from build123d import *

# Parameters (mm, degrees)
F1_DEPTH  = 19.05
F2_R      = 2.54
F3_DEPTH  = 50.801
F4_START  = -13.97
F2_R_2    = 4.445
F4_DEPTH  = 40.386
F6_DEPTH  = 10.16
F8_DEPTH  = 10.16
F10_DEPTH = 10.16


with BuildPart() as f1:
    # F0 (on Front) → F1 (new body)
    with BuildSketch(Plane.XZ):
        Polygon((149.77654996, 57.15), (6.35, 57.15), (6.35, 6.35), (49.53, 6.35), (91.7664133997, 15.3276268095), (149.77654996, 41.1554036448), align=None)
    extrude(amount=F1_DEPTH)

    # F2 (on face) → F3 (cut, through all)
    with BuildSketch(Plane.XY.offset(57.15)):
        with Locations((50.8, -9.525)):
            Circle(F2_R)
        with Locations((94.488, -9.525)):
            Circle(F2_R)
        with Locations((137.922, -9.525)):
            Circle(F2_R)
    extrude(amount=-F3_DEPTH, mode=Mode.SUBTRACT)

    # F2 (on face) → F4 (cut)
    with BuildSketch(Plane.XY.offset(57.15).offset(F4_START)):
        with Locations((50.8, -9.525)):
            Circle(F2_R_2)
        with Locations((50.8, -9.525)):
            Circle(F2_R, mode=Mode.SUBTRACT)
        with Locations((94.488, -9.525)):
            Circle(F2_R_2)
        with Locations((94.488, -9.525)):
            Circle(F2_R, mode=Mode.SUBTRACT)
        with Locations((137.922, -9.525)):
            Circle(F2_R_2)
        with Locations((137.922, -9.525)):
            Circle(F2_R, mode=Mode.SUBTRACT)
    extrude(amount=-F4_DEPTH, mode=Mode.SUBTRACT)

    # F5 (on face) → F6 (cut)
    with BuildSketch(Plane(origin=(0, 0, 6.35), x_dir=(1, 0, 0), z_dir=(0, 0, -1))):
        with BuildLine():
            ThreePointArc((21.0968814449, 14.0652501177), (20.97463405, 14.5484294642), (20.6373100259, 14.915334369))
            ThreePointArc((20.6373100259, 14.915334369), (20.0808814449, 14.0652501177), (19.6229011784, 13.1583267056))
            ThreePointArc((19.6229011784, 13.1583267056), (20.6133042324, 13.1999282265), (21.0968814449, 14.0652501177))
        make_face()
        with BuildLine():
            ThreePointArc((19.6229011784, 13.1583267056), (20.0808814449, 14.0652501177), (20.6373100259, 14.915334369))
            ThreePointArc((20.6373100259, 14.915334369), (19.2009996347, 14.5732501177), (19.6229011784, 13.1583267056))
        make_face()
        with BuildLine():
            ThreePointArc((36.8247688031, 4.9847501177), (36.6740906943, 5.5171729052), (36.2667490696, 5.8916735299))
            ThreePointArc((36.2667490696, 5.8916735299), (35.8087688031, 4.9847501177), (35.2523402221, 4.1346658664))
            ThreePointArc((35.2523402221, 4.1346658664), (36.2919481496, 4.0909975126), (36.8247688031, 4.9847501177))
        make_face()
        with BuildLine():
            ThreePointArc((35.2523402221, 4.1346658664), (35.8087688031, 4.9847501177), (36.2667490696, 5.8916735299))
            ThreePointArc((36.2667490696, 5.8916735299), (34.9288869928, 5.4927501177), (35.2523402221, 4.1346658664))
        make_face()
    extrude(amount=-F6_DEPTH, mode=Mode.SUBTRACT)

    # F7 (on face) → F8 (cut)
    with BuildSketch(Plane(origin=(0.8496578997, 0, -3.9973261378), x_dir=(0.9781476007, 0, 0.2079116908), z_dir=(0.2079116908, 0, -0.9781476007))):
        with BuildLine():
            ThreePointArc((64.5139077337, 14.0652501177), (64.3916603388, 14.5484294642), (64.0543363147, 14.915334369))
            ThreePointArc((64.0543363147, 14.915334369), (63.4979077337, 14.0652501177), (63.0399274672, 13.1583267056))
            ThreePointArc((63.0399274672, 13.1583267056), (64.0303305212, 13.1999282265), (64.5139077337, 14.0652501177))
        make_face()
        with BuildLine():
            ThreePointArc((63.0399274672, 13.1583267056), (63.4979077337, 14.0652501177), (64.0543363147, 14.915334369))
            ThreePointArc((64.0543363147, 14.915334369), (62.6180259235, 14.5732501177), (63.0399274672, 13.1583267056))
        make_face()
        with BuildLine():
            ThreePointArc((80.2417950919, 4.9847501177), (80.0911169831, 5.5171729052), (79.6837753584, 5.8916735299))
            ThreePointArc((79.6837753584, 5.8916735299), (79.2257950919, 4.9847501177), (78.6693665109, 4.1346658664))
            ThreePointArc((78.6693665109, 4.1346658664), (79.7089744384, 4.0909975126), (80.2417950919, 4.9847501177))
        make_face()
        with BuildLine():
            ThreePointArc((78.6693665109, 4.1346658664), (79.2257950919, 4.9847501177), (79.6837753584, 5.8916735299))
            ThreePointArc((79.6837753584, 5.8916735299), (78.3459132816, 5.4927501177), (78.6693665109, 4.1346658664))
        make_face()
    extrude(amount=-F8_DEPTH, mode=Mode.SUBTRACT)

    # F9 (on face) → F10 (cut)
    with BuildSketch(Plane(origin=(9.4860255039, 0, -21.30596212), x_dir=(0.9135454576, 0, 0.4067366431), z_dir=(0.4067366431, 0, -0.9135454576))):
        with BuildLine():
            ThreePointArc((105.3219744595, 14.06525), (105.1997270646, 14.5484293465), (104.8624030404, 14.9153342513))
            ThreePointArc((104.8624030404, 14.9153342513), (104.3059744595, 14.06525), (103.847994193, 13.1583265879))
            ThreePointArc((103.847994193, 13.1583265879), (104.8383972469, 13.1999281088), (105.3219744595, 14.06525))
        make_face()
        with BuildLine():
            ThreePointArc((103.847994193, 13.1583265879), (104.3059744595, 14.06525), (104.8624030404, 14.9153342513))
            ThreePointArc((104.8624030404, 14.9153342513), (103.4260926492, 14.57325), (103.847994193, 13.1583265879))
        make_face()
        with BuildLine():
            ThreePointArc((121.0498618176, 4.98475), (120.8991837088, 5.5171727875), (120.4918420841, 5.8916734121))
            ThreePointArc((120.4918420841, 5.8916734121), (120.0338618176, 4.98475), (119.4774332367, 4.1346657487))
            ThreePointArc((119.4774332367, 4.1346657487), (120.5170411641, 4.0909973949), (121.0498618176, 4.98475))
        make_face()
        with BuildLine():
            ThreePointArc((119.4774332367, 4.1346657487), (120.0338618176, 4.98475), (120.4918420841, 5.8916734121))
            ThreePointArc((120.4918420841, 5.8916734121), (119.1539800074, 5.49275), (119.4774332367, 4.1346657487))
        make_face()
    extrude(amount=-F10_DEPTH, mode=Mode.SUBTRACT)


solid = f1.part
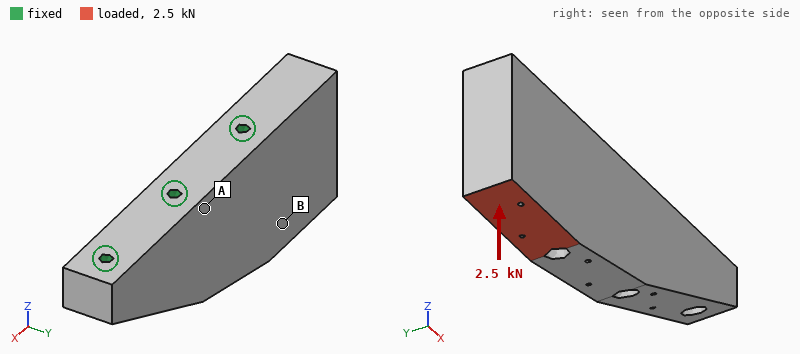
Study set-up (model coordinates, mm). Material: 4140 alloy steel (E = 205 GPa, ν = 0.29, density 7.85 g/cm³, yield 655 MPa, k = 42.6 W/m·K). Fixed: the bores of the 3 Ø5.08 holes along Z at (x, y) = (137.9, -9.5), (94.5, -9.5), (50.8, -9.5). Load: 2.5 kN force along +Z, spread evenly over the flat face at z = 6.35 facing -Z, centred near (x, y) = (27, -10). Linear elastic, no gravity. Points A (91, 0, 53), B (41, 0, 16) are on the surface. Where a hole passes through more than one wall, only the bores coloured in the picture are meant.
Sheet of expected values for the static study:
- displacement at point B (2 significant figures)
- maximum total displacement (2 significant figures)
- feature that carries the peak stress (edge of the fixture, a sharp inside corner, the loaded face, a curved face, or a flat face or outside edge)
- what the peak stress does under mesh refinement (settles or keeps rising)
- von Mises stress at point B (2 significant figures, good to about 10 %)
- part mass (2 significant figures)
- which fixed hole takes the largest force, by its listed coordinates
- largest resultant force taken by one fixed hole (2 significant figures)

2.6 µm
5.6 µm
edge of the fixture
keeps rising
6.4 MPa
830 g
(50.8, -9.5)
3.3 kN
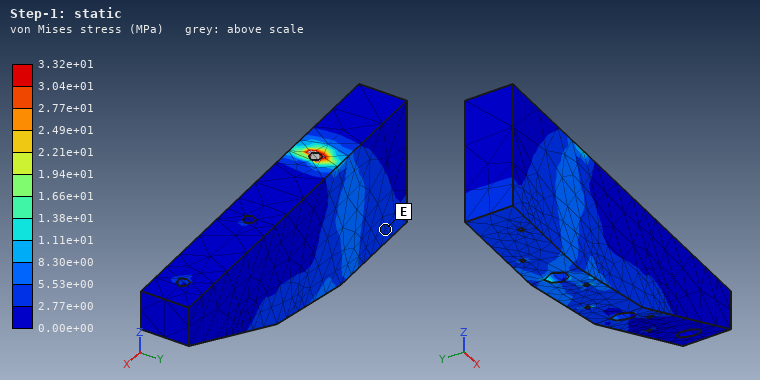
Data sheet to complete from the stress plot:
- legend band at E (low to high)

2.77e+00 to 5.53e+00 MPa
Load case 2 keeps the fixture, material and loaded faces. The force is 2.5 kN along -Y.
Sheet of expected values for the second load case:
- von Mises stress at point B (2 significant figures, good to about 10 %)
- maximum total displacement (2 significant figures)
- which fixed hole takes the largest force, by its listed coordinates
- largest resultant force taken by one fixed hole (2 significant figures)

16 MPa
47 µm
(50.8, -9.5)
3.3 kN
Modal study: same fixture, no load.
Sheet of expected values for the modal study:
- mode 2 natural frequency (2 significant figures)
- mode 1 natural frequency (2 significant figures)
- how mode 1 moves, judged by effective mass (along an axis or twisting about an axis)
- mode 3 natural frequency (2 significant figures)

6000 Hz
3500 Hz
along Y
6900 Hz
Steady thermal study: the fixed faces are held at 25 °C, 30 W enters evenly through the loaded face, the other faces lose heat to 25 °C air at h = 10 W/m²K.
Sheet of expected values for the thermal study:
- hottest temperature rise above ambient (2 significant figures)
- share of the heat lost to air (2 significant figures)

46 K
8.0 %
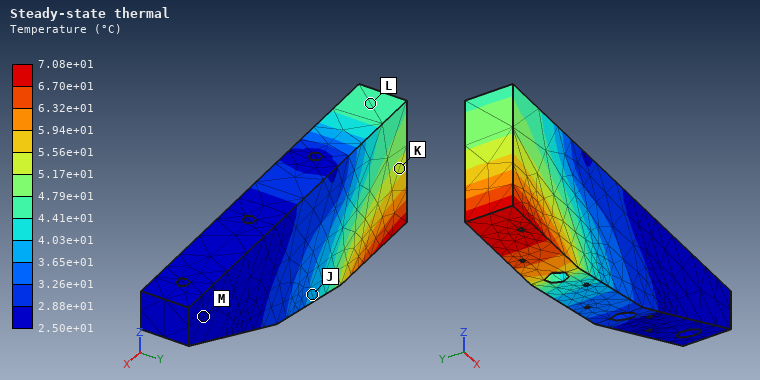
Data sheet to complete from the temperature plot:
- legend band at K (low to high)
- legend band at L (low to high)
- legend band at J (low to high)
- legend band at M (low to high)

5.17e+01 to 5.56e+01 °C
4.41e+01 to 4.79e+01 °C
3.65e+01 to 4.03e+01 °C
2.50e+01 to 2.88e+01 °C
